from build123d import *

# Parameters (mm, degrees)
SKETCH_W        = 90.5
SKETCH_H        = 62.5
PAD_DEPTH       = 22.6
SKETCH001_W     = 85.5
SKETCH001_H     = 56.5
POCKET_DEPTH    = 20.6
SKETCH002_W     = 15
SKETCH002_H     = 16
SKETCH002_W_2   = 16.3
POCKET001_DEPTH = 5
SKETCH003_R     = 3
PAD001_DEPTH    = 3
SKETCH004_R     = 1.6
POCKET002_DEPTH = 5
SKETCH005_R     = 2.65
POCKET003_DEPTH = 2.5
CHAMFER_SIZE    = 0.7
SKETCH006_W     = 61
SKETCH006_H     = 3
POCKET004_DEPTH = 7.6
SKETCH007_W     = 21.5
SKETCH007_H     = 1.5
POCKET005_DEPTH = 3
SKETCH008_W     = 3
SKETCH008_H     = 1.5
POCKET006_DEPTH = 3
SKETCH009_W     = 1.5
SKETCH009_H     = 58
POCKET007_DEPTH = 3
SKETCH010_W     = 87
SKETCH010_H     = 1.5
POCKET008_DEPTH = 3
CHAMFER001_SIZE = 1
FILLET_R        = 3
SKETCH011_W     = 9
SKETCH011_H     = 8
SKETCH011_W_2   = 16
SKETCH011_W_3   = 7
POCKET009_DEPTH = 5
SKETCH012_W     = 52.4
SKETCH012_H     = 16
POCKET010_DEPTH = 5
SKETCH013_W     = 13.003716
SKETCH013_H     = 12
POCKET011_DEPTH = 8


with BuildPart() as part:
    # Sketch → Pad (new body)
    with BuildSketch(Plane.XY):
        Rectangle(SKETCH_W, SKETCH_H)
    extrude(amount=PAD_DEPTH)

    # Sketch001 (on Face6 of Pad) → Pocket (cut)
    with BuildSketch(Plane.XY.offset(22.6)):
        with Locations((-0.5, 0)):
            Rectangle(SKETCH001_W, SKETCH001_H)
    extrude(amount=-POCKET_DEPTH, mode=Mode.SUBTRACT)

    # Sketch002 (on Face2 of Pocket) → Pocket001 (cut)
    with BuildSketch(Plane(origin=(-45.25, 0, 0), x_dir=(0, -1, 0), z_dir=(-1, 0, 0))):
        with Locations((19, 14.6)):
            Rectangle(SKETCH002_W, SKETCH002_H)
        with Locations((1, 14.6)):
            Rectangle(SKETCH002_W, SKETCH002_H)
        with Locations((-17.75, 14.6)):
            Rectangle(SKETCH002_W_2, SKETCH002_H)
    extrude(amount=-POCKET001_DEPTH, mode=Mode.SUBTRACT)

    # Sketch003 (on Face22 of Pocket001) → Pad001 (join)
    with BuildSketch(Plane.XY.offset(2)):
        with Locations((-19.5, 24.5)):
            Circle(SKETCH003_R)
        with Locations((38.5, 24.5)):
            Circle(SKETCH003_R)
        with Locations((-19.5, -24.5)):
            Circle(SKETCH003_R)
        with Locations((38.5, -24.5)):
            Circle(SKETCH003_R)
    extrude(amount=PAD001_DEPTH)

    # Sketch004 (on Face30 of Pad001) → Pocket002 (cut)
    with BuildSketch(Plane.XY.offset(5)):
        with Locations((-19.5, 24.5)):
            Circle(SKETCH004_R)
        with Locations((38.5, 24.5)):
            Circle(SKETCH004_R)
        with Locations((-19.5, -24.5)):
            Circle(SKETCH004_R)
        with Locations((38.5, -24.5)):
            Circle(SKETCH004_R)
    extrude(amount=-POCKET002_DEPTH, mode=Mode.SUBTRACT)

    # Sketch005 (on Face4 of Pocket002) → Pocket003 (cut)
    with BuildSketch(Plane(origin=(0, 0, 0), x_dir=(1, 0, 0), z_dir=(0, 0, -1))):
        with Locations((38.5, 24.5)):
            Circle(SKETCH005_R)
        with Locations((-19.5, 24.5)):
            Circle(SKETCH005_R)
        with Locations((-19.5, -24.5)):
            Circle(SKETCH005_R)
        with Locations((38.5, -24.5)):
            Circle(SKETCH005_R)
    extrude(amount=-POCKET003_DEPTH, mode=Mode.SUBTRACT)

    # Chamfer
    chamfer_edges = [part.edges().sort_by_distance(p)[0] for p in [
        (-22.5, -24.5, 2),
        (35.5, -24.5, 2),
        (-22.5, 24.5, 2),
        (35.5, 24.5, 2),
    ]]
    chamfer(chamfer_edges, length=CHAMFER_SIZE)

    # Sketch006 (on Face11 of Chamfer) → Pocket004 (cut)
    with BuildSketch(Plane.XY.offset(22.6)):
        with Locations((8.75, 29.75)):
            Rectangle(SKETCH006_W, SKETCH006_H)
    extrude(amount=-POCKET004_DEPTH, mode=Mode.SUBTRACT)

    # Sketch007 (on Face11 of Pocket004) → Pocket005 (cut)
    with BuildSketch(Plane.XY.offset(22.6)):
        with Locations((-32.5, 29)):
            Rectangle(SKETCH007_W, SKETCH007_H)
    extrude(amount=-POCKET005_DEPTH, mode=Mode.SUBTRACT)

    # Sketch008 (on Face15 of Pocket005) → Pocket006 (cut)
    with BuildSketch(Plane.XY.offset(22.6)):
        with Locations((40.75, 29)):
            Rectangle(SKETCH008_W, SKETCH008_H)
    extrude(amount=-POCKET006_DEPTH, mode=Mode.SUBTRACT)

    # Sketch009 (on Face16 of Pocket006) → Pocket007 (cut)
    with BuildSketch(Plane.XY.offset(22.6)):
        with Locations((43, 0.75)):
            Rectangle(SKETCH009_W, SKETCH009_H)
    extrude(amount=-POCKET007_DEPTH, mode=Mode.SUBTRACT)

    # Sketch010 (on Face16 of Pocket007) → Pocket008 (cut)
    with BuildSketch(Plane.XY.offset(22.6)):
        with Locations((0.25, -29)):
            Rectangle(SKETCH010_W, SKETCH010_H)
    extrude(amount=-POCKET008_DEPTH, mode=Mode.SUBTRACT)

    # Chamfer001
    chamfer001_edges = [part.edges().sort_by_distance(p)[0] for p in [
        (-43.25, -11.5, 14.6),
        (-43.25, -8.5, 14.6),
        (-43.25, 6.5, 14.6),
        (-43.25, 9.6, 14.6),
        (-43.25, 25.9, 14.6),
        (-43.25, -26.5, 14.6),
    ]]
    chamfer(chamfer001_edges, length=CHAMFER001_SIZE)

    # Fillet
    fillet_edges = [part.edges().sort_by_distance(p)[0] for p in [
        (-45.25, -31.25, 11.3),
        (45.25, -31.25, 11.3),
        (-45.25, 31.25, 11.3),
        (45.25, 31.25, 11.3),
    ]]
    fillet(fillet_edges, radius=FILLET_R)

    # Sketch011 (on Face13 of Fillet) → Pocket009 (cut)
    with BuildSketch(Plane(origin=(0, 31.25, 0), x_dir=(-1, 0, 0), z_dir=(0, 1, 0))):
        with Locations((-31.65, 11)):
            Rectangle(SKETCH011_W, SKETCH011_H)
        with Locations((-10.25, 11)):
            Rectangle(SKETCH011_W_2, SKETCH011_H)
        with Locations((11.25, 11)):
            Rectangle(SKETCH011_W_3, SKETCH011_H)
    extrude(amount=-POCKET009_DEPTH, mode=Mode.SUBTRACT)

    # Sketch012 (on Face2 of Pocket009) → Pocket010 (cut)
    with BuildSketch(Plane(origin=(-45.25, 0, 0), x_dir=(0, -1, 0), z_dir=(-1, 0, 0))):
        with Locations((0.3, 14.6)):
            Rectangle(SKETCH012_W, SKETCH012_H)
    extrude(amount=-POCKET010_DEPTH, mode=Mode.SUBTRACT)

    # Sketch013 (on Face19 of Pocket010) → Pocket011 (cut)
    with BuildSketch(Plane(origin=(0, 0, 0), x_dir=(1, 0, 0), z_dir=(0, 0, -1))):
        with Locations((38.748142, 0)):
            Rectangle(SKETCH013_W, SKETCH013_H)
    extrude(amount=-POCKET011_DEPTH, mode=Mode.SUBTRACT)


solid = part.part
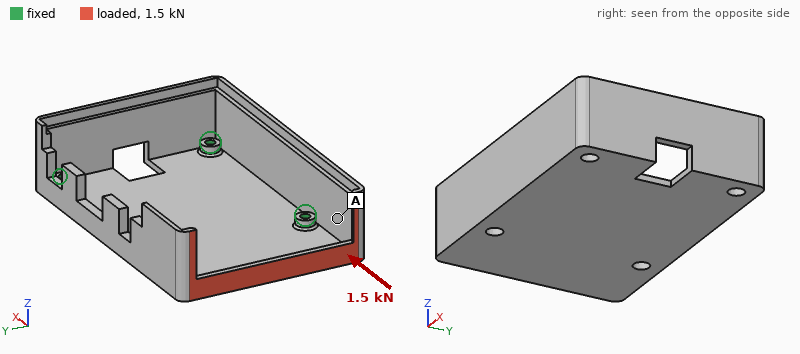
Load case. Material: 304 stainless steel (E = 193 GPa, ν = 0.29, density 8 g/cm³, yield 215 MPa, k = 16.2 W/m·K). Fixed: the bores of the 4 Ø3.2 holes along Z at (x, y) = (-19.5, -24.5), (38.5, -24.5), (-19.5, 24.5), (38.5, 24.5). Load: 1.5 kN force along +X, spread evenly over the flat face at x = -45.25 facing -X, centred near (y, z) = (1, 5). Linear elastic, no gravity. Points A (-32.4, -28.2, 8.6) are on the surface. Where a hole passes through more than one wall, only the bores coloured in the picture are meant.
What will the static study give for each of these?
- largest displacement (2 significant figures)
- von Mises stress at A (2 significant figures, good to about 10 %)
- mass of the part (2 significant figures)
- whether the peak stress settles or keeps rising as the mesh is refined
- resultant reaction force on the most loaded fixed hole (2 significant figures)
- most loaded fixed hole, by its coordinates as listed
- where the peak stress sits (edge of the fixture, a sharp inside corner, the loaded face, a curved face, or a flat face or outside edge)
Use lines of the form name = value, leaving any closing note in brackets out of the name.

largest displacement = 35 µm
von Mises stress at A = 9.0 MPa
mass of the part = 180 g
whether the peak stress settles or keeps rising as the mesh is refined = keeps rising
resultant reaction force on the most loaded fixed hole = 550 N
most loaded fixed hole, by its coordinates as listed = (-19.5, 24.5)
where the peak stress sits = edge of the fixture
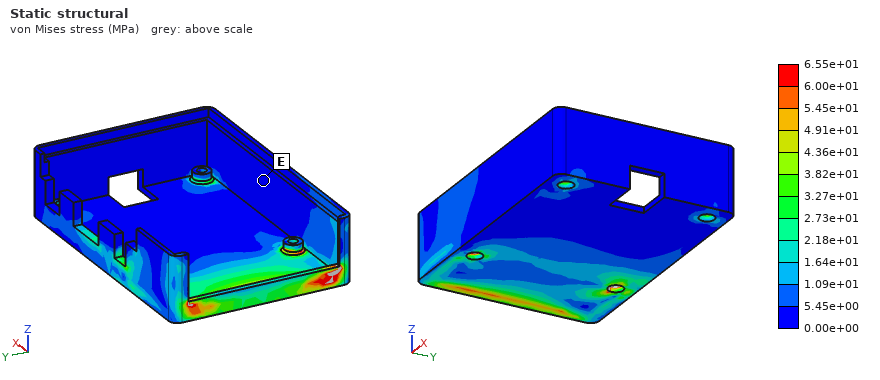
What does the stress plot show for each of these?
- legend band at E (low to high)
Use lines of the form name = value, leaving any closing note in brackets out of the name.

legend band at E = 0.00e+00 to 5.45e+00 MPa
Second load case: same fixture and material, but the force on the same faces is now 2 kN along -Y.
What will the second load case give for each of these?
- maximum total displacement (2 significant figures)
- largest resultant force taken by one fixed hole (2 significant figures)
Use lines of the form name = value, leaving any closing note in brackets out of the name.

maximum total displacement = 86 µm
largest resultant force taken by one fixed hole = 1.3 kN
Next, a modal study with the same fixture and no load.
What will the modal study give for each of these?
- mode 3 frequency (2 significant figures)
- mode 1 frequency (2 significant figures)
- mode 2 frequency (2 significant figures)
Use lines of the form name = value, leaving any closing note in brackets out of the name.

mode 3 frequency = 3600 Hz
mode 1 frequency = 2700 Hz
mode 2 frequency = 2800 Hz
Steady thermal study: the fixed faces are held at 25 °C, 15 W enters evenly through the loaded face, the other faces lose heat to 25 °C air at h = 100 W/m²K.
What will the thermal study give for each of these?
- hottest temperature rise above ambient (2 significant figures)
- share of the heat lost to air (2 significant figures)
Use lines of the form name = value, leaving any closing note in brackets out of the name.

hottest temperature rise above ambient = 72 K
share of the heat lost to air = 95 %
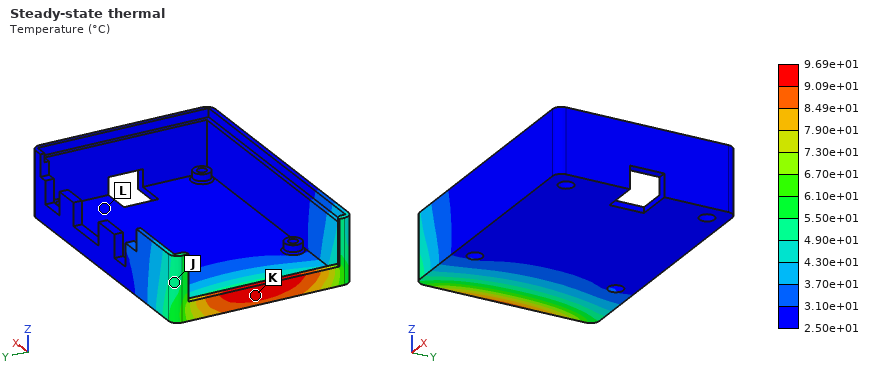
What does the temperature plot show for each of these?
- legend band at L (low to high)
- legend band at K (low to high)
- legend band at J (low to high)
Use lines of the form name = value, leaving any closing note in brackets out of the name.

legend band at L = 2.50e+01 to 3.10e+01 °C
legend band at K = 9.09e+01 to 9.69e+01 °C
legend band at J = 4.90e+01 to 5.50e+01 °C
